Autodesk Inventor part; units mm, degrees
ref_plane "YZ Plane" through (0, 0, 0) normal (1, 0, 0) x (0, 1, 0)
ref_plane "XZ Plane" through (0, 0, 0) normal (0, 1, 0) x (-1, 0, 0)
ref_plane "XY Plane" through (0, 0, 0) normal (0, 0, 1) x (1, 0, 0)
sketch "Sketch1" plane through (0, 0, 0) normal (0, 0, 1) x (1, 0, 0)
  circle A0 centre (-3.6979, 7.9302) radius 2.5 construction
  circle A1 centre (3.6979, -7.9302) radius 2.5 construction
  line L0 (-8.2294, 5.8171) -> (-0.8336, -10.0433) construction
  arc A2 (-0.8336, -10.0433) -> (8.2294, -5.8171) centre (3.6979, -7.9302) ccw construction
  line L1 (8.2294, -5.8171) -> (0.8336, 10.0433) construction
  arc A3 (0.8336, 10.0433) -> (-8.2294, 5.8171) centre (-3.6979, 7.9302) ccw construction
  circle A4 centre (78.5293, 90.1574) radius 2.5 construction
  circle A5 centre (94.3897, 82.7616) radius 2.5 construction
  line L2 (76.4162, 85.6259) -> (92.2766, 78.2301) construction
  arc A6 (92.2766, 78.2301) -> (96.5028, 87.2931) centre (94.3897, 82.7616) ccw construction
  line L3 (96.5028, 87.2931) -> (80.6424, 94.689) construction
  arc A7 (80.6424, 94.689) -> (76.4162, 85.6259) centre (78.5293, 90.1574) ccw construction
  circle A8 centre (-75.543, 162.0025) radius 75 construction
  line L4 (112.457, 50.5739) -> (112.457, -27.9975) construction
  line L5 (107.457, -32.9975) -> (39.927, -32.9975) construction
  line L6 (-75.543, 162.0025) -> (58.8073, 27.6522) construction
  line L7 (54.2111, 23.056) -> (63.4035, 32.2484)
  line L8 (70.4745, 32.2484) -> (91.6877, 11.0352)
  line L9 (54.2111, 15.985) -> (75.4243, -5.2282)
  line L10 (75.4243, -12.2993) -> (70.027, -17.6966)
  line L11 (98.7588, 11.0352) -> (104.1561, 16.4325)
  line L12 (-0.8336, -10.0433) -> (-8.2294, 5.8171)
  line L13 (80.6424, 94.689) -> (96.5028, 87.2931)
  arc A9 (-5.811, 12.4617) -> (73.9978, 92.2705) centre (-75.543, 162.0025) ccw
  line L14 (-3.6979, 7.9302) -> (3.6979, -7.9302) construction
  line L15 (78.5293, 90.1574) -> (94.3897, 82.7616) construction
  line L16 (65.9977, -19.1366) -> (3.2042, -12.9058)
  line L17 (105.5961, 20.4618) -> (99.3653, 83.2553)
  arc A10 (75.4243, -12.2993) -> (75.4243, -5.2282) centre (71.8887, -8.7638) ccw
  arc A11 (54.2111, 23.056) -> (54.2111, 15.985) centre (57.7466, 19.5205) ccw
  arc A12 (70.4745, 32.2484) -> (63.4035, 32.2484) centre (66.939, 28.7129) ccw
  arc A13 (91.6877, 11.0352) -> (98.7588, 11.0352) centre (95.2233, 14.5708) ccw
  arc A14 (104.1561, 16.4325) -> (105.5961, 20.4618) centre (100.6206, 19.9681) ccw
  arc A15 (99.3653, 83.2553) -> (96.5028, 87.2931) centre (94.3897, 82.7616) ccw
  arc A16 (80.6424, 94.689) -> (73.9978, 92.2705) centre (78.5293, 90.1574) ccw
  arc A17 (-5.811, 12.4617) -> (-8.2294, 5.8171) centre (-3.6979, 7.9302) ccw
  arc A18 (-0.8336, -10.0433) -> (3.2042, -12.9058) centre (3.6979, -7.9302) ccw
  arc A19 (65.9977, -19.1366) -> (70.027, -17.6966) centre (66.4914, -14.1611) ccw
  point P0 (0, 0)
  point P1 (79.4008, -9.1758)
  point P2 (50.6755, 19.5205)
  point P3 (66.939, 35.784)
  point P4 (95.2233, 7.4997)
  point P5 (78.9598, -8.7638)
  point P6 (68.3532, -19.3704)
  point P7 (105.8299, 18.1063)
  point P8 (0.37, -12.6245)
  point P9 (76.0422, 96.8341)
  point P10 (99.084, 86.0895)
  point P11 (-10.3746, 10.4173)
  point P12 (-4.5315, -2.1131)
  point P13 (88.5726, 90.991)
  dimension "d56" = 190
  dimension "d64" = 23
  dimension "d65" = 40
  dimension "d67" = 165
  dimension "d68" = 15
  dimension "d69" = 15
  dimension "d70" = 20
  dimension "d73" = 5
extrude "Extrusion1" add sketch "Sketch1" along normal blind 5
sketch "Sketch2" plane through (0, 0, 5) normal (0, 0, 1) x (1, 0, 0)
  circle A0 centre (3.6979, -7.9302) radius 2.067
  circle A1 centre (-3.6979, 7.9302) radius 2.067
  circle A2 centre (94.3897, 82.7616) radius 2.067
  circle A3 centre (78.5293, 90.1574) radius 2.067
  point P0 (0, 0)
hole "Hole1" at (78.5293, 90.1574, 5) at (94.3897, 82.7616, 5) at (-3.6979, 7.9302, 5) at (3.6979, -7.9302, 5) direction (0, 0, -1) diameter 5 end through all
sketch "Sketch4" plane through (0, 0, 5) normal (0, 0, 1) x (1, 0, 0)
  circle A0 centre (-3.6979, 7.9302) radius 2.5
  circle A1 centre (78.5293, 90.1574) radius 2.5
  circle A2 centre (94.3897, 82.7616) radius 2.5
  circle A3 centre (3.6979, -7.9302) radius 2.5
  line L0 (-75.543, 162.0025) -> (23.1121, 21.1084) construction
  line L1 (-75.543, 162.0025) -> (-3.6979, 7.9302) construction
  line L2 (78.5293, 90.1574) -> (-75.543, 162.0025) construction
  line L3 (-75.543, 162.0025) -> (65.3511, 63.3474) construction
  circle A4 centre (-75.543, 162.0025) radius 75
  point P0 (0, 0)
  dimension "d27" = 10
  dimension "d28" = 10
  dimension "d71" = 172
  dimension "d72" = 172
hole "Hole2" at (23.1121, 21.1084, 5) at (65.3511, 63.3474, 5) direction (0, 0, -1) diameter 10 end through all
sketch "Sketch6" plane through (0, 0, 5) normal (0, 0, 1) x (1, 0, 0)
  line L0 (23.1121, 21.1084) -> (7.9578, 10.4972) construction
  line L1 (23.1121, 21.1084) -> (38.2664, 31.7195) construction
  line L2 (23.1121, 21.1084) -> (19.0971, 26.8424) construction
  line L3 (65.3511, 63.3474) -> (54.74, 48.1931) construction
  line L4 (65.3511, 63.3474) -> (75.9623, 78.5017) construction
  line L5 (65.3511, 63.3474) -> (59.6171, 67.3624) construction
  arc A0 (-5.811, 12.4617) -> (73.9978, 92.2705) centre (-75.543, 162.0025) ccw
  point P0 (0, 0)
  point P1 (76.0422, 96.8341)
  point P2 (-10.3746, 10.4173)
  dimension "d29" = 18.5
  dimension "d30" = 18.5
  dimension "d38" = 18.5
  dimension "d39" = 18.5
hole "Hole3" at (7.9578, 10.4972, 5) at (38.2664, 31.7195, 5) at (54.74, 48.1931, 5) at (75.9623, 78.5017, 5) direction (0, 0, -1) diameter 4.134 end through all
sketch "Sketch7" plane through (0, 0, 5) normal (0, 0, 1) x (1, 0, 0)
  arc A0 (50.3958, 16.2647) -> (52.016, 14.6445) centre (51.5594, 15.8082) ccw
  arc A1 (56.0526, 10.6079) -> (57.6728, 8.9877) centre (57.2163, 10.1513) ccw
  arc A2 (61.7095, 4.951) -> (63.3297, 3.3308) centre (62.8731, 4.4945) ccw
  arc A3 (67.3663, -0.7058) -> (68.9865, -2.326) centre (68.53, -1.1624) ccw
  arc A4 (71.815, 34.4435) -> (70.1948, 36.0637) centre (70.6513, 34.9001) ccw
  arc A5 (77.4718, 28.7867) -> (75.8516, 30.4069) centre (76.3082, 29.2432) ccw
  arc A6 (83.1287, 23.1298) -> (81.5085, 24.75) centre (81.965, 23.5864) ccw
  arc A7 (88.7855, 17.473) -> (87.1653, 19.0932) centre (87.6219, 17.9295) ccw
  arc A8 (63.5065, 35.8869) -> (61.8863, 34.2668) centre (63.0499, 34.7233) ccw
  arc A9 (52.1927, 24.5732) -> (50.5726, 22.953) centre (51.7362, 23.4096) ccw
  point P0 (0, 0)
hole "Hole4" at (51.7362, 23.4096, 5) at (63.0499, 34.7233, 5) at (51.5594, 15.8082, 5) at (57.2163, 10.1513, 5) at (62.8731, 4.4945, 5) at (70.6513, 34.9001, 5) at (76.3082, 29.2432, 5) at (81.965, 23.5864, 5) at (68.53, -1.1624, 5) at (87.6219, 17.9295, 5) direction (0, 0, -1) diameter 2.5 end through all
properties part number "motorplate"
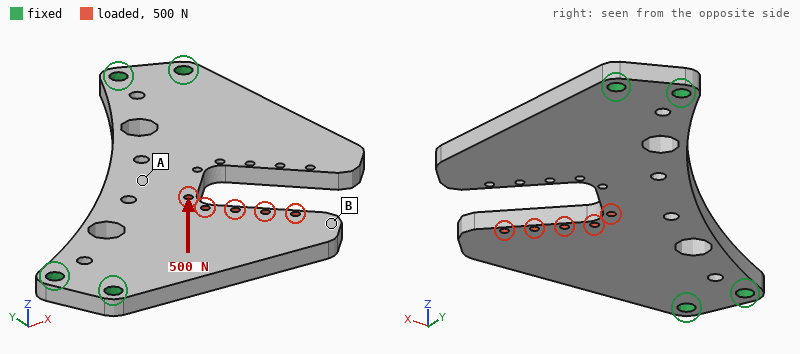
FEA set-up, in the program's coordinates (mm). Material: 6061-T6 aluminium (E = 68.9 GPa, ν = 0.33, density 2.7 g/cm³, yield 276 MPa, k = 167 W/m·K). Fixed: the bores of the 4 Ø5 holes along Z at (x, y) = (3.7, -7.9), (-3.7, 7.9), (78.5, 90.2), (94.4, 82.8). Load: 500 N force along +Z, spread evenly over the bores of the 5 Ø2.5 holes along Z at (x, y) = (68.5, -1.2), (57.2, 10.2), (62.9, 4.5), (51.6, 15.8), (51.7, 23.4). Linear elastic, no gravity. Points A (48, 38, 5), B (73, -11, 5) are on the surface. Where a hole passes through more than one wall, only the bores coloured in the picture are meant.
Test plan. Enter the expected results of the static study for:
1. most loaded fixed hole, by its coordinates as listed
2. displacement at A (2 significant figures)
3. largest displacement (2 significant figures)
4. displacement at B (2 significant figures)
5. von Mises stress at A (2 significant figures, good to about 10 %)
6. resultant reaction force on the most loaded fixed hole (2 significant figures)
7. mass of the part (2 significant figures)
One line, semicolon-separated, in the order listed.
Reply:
(3.7, -7.9); 0.22 mm; 0.89 mm; 0.83 mm; 49 MPa; 500 N; 81 g
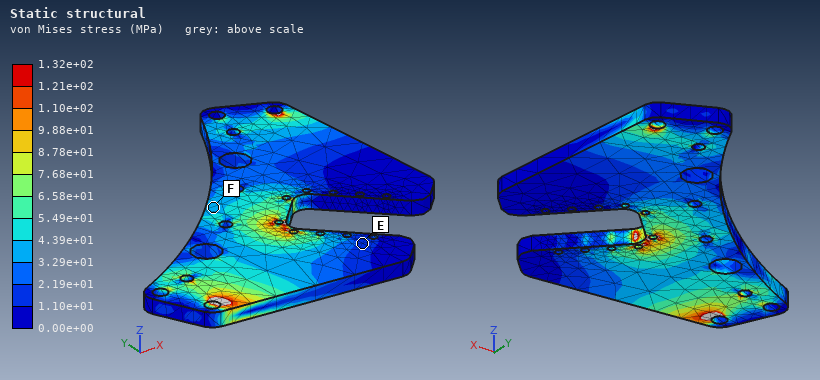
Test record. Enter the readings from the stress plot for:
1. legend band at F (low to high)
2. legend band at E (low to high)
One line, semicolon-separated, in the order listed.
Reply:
3.29e+01 to 4.39e+01 MPa; 1.10e+01 to 2.19e+01 MPa
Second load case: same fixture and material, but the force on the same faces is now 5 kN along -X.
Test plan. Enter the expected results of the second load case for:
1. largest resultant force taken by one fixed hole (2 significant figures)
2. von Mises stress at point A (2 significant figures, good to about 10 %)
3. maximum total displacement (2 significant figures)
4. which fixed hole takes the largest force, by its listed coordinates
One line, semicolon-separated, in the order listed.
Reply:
3.1 kN; 10 MPa; 66 µm; (-3.7, 7.9)
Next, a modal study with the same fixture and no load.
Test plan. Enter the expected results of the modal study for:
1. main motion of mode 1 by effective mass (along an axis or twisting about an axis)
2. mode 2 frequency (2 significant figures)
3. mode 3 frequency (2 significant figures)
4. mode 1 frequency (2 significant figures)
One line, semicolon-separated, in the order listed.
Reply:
along Z; 1500 Hz; 2300 Hz; 940 Hz
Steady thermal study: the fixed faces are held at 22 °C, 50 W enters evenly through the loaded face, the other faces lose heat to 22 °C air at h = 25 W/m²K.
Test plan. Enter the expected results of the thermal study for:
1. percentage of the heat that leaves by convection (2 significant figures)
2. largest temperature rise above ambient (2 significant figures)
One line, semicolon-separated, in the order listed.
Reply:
18 %; 72 K
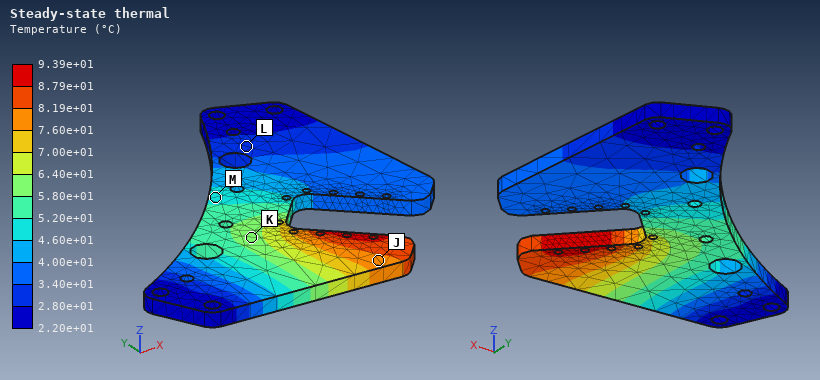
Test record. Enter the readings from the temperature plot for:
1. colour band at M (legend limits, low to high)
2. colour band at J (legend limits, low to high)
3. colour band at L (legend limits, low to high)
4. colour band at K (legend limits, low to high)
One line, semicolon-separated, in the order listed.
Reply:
4.60e+01 to 5.20e+01 °C; 7.60e+01 to 8.19e+01 °C; 2.80e+01 to 3.40e+01 °C; 5.80e+01 to 6.40e+01 °C
